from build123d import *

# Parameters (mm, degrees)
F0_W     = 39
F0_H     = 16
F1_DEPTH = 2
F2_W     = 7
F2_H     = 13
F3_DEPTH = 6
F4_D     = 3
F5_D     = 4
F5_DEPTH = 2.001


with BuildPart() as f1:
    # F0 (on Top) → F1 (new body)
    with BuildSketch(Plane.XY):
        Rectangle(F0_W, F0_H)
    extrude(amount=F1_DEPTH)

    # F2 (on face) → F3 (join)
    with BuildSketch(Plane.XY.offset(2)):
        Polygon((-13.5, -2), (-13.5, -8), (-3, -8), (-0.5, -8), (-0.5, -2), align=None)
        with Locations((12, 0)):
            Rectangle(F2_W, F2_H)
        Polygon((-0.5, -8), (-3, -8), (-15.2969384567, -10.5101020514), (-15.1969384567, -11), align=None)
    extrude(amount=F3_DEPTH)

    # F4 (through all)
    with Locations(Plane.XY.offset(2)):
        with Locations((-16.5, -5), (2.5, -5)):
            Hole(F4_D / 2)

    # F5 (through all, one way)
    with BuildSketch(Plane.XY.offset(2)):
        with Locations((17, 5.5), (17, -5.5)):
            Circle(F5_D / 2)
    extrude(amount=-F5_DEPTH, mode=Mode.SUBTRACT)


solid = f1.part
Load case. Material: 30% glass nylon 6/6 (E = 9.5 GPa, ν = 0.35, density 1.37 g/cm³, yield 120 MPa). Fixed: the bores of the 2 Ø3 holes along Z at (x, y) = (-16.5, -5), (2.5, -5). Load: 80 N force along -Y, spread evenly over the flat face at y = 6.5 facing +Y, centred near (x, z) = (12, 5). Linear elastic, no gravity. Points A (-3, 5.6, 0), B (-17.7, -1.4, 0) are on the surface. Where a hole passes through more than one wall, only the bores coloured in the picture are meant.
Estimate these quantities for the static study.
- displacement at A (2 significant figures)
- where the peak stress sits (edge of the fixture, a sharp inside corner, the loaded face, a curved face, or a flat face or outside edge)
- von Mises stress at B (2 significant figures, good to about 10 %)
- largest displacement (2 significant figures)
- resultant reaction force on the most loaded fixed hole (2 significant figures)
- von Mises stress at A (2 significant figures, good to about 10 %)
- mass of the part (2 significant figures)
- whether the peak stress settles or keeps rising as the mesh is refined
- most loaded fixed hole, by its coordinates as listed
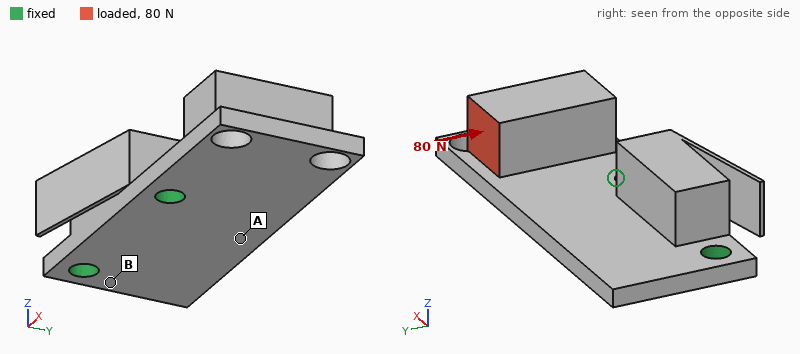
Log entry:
0.045 mm
edge of the fixture
4.4 MPa
0.19 mm
110 N
12 MPa
3.0 g
keeps rising
(2.5, -5)
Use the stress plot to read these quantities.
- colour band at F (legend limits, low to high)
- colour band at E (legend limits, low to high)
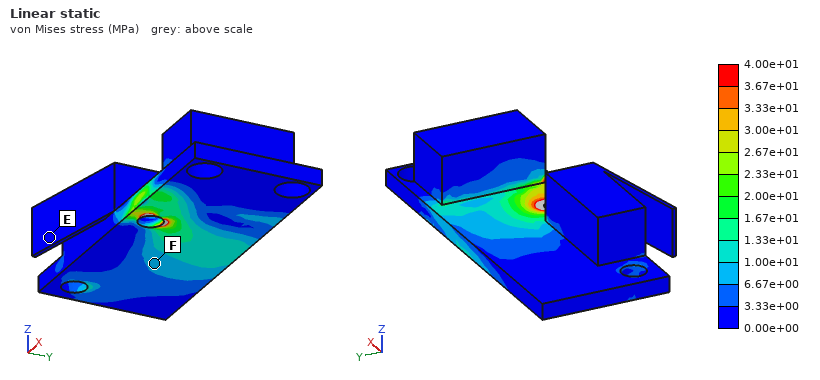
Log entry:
6.67e+00 to 1.00e+01 MPa
0.00e+00 to 3.33e+00 MPa
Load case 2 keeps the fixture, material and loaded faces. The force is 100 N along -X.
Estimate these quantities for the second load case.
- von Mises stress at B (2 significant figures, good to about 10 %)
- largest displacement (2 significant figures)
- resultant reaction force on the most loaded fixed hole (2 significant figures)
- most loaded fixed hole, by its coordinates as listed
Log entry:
6.8 MPa
0.44 mm
77 N
(-16.5, -5)
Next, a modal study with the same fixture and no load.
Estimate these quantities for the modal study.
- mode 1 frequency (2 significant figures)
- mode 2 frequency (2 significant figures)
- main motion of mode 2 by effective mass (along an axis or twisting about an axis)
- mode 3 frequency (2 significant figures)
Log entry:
1300 Hz
1900 Hz
along Z
3900 Hz
